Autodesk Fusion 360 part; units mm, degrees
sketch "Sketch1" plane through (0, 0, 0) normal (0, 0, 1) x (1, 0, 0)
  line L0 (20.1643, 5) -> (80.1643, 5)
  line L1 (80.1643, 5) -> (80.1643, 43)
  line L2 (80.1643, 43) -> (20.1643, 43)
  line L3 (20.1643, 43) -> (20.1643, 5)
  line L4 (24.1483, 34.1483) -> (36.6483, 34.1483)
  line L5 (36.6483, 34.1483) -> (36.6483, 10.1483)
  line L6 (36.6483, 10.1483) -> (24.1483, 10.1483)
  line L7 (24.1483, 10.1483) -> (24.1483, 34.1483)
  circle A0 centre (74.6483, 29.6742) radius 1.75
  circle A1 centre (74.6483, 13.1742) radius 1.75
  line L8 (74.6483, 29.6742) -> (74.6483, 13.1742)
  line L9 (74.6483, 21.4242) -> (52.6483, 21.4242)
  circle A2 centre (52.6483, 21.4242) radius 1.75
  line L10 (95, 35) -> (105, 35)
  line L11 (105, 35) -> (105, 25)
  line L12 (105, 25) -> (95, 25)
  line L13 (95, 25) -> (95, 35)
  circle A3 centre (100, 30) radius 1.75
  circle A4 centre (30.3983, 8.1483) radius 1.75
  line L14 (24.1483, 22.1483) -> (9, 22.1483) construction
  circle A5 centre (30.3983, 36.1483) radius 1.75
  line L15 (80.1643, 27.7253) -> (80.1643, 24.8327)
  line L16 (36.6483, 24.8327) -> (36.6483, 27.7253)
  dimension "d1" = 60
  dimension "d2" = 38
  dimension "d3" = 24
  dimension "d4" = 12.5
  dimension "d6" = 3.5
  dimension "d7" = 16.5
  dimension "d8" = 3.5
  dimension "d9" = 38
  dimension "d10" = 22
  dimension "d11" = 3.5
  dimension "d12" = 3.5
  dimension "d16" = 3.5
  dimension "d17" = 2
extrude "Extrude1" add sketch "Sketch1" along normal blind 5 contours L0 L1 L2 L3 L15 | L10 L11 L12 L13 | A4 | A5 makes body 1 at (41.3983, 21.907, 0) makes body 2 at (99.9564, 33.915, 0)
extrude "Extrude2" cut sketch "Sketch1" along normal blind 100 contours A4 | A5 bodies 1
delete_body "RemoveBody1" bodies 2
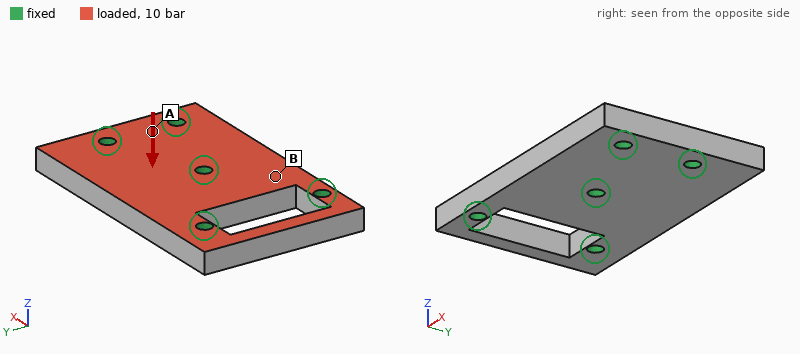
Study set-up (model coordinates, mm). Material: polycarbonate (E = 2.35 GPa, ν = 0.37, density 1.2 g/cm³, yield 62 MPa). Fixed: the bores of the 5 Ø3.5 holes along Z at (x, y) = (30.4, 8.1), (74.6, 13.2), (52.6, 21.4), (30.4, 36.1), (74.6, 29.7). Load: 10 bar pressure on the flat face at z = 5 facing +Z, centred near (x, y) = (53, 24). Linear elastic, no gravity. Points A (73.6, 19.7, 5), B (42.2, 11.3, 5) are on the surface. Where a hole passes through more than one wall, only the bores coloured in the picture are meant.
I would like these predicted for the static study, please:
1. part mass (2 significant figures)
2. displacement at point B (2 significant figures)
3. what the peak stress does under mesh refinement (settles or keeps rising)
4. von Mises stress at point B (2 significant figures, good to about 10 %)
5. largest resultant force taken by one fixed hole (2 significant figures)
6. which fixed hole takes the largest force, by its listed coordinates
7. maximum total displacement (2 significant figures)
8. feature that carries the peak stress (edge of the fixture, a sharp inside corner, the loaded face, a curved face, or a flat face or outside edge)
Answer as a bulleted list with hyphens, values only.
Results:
- 12 g
- 0.11 mm
- keeps rising
- 9.4 MPa
- 690 N
- (52.6, 21.4)
- 0.47 mm
- edge of the fixture
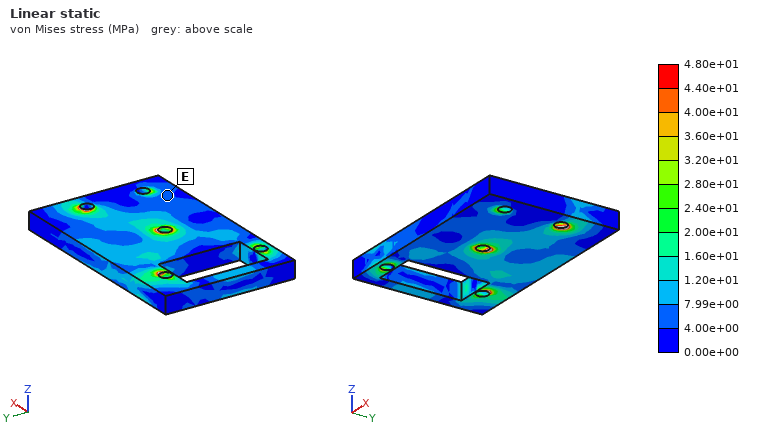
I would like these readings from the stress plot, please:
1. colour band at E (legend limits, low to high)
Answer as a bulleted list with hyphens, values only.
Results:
- 4.00e+00 to 7.99e+00 MPa
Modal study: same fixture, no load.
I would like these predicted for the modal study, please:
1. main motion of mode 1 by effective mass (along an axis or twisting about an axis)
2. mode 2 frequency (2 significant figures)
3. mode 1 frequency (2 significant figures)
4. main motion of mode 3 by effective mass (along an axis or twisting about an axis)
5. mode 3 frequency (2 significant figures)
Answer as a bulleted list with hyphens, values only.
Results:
- along Z
- 4700 Hz
- 3900 Hz
- along Z
- 5500 Hz
